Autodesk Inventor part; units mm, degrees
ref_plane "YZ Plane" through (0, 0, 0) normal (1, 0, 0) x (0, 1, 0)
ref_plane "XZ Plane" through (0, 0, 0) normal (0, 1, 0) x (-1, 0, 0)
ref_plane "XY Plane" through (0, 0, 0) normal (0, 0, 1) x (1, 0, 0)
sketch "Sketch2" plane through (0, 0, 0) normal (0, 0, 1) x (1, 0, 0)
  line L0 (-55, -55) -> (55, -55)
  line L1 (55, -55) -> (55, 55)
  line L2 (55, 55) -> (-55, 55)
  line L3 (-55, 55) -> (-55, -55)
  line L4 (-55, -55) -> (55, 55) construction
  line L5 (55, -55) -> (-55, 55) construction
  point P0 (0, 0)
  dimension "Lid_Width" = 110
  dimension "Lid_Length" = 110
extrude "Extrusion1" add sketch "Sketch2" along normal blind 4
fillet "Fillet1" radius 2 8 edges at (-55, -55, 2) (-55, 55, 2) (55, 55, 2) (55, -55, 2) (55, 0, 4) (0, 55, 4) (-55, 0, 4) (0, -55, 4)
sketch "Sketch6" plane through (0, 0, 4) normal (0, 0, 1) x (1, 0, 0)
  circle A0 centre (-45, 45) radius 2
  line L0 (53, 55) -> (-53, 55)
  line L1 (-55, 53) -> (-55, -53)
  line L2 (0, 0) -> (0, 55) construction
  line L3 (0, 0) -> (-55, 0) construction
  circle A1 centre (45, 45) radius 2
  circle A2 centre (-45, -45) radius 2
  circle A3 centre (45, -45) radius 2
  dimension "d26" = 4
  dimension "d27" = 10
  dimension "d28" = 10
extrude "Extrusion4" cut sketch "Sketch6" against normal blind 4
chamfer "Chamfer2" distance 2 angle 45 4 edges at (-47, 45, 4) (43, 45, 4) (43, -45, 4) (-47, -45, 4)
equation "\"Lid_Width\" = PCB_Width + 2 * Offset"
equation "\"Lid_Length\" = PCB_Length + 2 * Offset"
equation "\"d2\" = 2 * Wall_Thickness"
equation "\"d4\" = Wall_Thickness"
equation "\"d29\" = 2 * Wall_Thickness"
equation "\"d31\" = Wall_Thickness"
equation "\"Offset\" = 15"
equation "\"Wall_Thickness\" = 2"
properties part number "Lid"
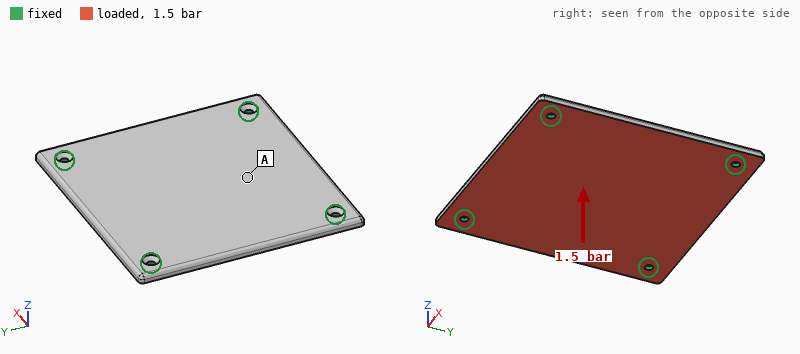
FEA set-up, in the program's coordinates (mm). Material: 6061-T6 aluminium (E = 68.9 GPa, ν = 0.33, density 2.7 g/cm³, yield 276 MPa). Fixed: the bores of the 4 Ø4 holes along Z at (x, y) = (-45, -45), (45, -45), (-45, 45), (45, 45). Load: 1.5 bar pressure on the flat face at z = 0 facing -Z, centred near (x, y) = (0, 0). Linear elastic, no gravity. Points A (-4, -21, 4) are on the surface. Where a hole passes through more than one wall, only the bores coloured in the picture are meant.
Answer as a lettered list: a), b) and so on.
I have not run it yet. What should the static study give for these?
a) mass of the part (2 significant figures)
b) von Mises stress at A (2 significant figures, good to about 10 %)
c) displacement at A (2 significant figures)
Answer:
a) 130 g
b) 28 MPa
c) 0.21 mm
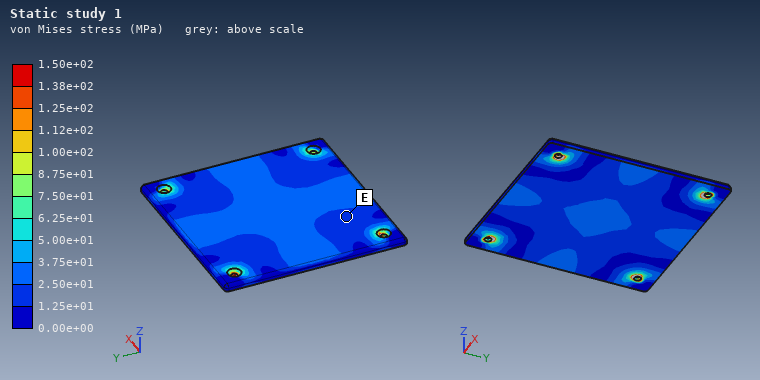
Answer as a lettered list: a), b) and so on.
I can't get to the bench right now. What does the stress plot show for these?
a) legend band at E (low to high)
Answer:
a) 1.25e+01 to 2.50e+01 MPa
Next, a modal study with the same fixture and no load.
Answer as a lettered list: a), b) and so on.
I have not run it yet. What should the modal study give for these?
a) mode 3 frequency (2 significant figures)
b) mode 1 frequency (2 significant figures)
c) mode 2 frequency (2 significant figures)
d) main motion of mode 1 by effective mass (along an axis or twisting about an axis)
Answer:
a) 2500 Hz
b) 1500 Hz
c) 2500 Hz
d) along Z
